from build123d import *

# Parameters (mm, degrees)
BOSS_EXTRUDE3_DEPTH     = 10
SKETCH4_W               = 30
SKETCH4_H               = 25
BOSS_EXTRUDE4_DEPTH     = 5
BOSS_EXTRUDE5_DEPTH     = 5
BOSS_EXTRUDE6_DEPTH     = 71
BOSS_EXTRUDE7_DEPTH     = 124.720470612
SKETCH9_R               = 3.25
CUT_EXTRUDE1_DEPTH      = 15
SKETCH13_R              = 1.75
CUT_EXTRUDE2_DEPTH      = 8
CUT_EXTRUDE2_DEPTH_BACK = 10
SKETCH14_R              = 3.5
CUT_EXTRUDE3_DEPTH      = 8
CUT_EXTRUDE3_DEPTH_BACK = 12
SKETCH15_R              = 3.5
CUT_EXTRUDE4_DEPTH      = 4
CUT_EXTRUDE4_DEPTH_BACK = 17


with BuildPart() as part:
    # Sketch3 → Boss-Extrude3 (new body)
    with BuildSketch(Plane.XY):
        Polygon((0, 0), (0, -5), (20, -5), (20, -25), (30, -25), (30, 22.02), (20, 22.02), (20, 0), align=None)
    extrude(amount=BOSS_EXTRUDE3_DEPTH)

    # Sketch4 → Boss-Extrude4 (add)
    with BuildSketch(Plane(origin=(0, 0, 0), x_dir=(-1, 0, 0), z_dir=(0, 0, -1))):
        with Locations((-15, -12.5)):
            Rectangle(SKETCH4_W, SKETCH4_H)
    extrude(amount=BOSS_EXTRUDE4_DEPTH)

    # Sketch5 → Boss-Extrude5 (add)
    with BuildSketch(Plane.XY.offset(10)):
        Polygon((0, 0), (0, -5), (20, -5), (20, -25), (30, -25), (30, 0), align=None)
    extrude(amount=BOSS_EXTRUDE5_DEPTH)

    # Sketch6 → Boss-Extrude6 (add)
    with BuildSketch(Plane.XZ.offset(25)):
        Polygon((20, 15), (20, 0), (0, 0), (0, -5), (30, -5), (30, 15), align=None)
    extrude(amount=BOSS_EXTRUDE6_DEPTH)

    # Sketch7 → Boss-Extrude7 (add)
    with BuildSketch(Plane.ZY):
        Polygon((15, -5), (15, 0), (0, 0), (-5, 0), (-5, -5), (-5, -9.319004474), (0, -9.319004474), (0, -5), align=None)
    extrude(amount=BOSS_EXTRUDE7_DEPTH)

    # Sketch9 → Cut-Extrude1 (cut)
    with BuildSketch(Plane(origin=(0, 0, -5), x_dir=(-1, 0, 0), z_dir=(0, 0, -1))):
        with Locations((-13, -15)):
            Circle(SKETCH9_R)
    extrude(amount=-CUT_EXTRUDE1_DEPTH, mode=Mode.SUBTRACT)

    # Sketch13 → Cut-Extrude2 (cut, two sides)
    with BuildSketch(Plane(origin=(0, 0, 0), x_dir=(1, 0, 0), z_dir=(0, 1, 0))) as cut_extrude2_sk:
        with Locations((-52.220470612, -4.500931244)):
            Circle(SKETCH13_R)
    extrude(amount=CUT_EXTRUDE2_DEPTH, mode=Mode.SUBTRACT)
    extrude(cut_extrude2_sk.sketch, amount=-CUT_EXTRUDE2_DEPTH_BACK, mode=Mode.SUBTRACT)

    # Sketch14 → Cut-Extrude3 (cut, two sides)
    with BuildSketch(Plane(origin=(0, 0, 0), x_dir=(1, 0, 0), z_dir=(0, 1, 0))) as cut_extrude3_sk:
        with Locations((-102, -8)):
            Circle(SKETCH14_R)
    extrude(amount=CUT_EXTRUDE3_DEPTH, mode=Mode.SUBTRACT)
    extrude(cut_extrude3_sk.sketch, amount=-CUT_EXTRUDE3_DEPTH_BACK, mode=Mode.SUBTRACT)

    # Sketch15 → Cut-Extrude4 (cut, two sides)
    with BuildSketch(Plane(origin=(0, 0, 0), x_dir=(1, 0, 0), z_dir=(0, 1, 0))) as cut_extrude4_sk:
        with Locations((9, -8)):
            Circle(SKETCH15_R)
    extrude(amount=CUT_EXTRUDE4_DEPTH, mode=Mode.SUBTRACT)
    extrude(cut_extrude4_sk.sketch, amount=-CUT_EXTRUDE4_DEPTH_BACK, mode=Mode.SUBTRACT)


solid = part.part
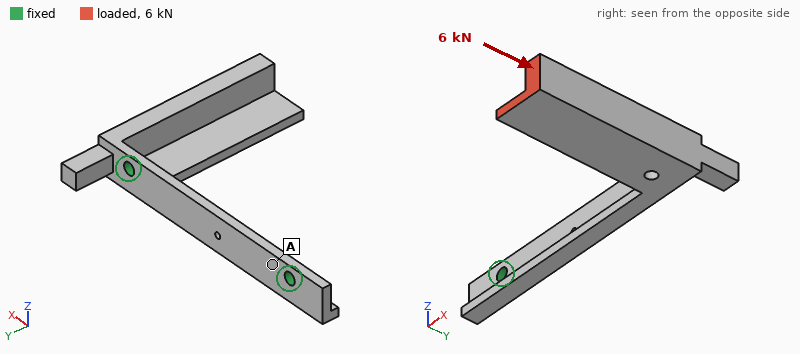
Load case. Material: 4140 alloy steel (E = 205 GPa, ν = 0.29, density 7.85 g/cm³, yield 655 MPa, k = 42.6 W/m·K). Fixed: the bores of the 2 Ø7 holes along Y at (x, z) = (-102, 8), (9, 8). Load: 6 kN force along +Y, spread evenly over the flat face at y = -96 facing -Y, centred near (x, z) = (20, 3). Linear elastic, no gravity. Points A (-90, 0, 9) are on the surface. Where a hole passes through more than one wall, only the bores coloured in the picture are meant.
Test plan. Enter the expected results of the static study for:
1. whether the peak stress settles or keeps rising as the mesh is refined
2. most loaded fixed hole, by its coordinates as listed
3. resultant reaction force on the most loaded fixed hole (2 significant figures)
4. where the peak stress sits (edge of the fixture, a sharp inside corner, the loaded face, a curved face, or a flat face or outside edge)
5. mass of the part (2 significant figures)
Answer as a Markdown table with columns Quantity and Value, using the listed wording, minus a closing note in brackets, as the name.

| Quantity | Value |
|---|---|
| whether the peak stress settles or keeps rising as the mesh is refined | keeps rising |
| most loaded fixed hole, by its coordinates as listed | (9, 8) |
| resultant reaction force on the most loaded fixed hole | 6.2 kN |
| where the peak stress sits | edge of the fixture |
| mass of the part | 370 g |
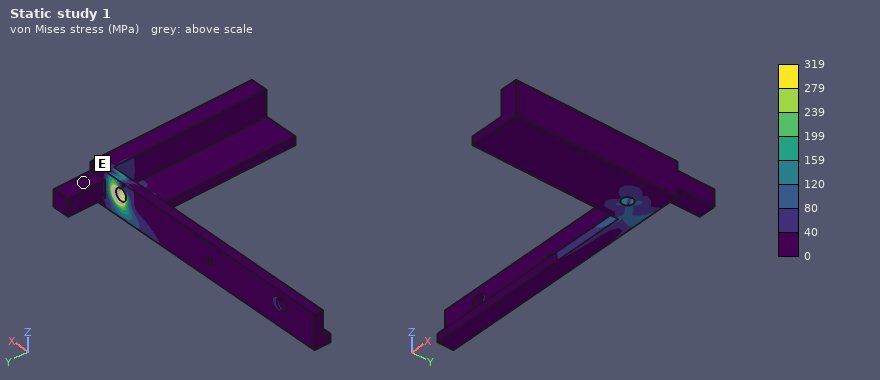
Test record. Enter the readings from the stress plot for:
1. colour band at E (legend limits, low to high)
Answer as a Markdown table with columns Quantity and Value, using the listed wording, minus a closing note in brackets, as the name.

| Quantity | Value |
|---|---|
| colour band at E | 0 to 40 MPa |
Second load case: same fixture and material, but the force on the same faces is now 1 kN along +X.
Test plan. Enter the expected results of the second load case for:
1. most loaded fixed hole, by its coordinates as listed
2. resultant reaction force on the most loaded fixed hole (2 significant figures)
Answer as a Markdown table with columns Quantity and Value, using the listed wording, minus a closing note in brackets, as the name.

| Quantity | Value |
|---|---|
| most loaded fixed hole, by its coordinates as listed | (-102, 8) |
| resultant reaction force on the most loaded fixed hole | 950 N |
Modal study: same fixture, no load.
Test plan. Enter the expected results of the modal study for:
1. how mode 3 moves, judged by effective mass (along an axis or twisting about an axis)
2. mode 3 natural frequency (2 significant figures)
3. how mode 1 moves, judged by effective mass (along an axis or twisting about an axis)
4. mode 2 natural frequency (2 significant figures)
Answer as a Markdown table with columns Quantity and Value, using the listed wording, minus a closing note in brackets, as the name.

| Quantity | Value |
|---|---|
| how mode 3 moves, judged by effective mass | along Y |
| mode 3 natural frequency | 3000 Hz |
| how mode 1 moves, judged by effective mass | along Z |
| mode 2 natural frequency | 870 Hz |
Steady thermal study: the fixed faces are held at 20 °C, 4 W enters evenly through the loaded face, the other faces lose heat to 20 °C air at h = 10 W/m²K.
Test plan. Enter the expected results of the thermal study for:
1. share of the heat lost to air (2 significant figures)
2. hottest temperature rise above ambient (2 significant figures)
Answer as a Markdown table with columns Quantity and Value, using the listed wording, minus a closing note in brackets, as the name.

| Quantity | Value |
|---|---|
| share of the heat lost to air | 37 % |
| hottest temperature rise above ambient | 27 K |
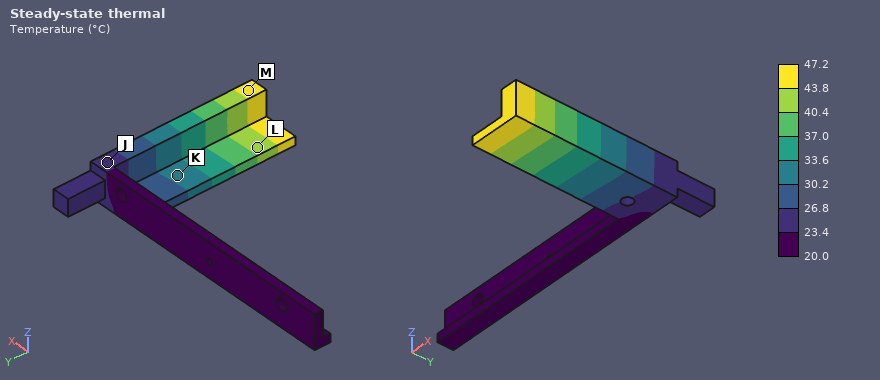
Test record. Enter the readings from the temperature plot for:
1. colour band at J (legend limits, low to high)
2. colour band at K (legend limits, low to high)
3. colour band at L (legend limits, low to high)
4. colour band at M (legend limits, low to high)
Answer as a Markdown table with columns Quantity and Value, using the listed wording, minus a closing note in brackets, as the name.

| Quantity | Value |
|---|---|
| colour band at J | 23.4 to 26.8 °C |
| colour band at K | 30.2 to 33.6 °C |
| colour band at L | 40.4 to 43.8 °C |
| colour band at M | 43.8 to 47.2 °C |
